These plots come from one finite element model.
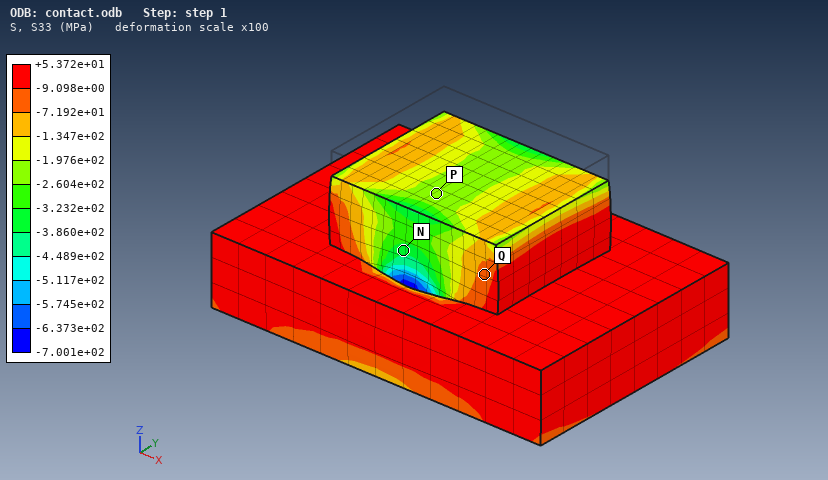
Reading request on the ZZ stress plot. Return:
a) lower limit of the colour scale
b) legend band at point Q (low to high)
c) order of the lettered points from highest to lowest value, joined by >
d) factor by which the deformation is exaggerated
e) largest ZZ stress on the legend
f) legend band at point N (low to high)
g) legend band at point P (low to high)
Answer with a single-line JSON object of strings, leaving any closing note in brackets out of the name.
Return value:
{"lower limit of the colour scale": "-7.001e+02 MPa", "legend band at point Q": "-7.192e+01 to -9.098e+00 MPa", "order of the lettered points from highest to lowest value, joined by >": "Q > P > N", "factor by which the deformation is exaggerated": "100", "largest ZZ stress on the legend": "+5.372e+01 MPa", "legend band at point N": "-3.860e+02 to -3.232e+02 MPa", "legend band at point P": "-2.604e+02 to -1.976e+02 MPa"}
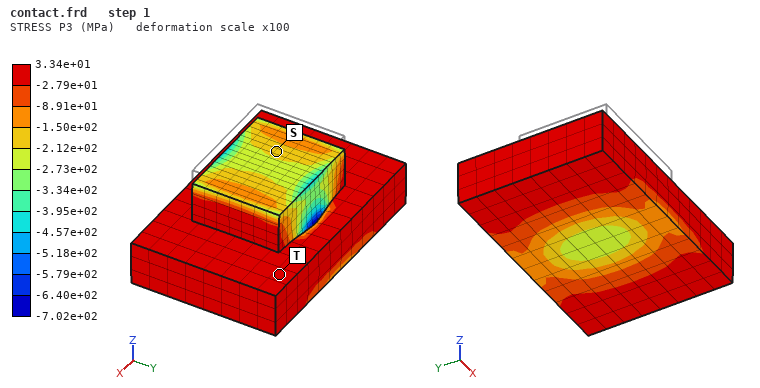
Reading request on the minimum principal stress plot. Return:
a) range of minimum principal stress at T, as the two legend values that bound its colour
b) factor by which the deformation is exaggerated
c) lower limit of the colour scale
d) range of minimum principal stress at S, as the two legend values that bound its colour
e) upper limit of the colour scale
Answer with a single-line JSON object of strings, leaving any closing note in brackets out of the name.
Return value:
{"range of minimum principal stress at T, as the two legend values that bound its colour": "-2.79e+01 to 3.34e+01 MPa", "factor by which the deformation is exaggerated": "100", "lower limit of the colour scale": "-7.02e+02 MPa", "range of minimum principal stress at S, as the two legend values that bound its colour": "-2.12e+02 to -1.50e+02 MPa", "upper limit of the colour scale": "3.34e+01 MPa"}
